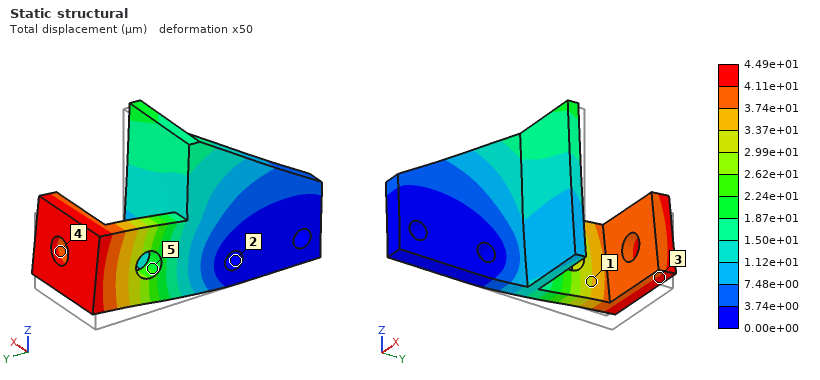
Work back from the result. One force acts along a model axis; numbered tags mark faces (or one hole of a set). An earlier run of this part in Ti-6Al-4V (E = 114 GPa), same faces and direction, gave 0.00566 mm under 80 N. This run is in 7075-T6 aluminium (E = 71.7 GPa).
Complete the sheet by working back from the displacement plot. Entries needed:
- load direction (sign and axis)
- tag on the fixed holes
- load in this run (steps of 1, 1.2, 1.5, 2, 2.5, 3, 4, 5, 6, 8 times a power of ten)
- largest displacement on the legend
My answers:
+Z
2
400 N
4.49e+01 µm
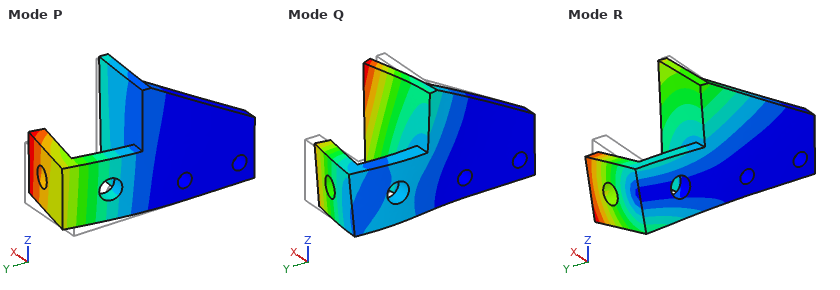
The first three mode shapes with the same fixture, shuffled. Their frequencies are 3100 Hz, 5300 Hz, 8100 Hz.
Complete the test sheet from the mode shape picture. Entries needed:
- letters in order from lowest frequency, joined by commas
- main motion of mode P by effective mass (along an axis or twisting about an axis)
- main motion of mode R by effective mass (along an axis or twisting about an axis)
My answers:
P, R, Q
along X
along Z
